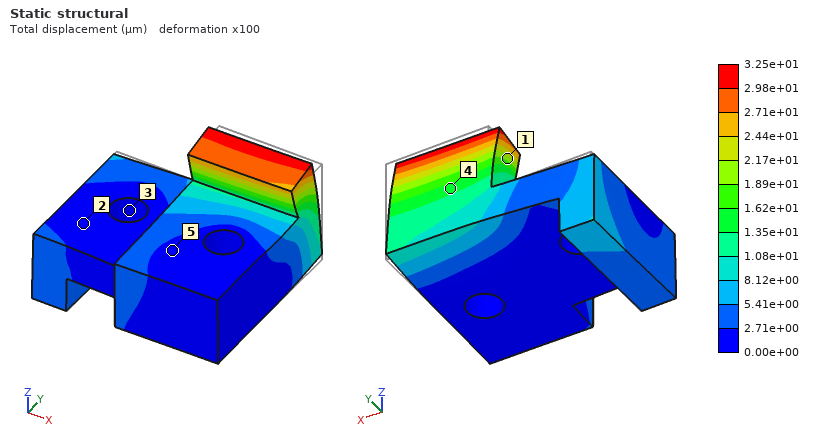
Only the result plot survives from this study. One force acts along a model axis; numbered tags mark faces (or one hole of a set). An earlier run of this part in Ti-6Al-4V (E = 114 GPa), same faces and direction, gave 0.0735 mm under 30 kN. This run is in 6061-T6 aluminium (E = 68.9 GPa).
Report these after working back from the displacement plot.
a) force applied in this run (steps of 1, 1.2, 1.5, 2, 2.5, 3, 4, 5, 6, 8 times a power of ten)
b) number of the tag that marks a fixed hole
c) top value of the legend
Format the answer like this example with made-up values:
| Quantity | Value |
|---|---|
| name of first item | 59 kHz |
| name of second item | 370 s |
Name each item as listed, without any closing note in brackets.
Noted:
| Quantity | Value |
|---|---|
| force applied in this run | 8 kN |
| number of the tag that marks a fixed hole | 3 |
| top value of the legend | 3.25e+01 µm |
